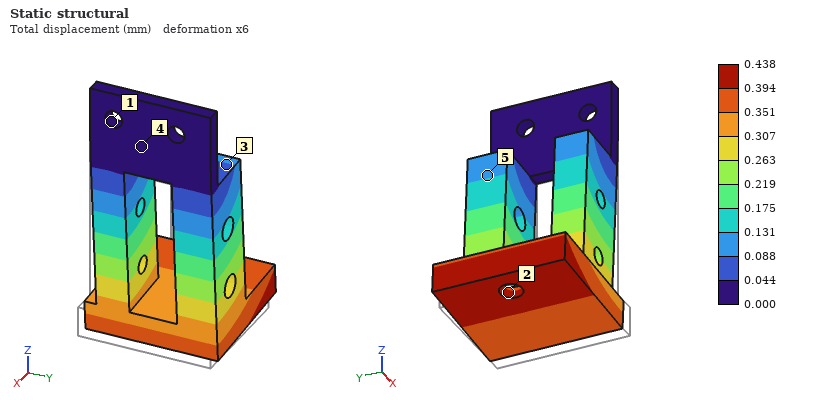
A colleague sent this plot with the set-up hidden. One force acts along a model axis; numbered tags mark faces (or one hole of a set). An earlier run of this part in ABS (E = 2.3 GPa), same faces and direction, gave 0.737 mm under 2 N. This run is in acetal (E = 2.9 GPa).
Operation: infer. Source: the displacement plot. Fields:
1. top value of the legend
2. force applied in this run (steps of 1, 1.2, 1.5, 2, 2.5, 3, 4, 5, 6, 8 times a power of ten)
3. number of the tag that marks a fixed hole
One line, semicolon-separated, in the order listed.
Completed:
0.438 mm; 1.5 N; 1
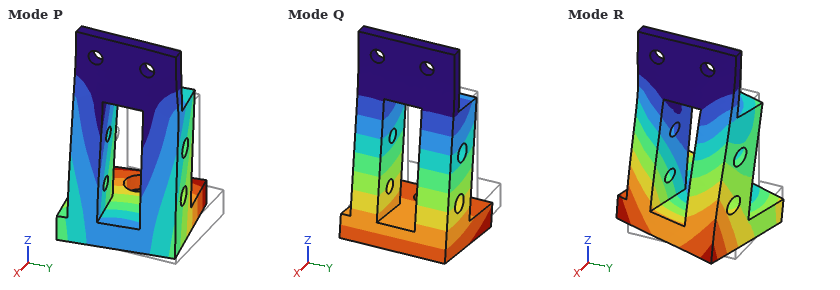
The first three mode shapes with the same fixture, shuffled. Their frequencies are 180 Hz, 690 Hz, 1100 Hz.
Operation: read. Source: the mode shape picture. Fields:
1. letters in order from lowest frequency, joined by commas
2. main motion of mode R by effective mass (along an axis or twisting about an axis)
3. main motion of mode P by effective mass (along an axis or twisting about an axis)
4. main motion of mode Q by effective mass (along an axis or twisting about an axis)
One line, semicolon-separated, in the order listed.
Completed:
Q, P, R; along Y; along Y; along X
